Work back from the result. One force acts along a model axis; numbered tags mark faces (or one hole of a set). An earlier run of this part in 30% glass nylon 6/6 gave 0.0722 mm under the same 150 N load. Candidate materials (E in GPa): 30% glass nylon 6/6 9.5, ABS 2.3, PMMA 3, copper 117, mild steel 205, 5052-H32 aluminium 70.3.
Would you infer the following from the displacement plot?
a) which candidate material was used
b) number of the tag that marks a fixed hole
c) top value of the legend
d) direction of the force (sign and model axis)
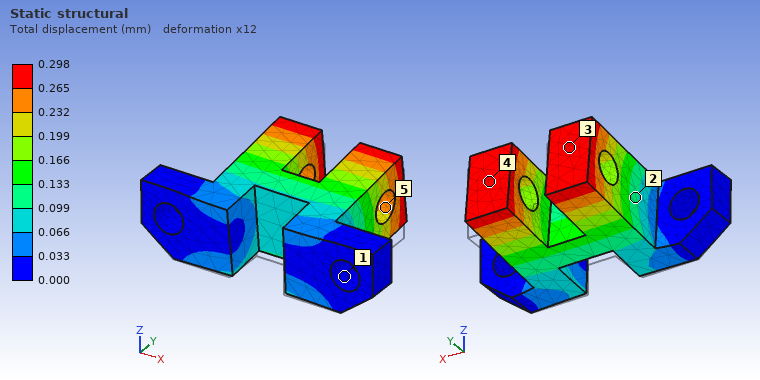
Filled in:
ABS
1
0.298 mm
+Z
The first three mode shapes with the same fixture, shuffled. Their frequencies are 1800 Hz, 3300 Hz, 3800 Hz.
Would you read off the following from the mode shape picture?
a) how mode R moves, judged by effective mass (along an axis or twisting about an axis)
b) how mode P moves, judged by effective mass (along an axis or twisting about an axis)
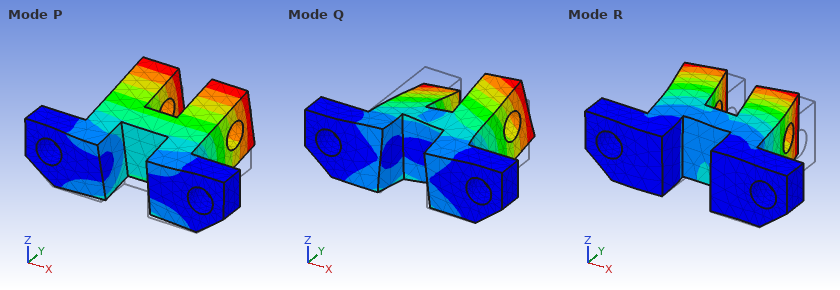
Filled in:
along X
along Z
